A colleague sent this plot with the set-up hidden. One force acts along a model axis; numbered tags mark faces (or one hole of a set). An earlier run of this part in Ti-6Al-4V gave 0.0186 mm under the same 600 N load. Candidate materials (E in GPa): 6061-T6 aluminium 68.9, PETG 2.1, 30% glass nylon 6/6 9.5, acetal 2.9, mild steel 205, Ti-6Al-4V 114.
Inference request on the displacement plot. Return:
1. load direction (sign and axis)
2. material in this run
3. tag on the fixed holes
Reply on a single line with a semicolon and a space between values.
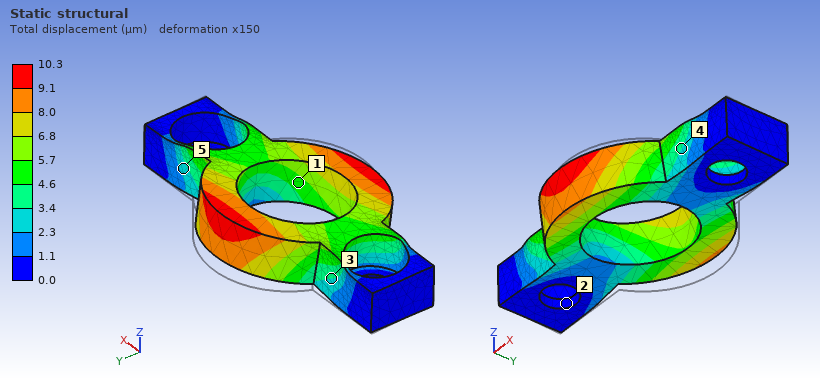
-Y; mild steel; 2
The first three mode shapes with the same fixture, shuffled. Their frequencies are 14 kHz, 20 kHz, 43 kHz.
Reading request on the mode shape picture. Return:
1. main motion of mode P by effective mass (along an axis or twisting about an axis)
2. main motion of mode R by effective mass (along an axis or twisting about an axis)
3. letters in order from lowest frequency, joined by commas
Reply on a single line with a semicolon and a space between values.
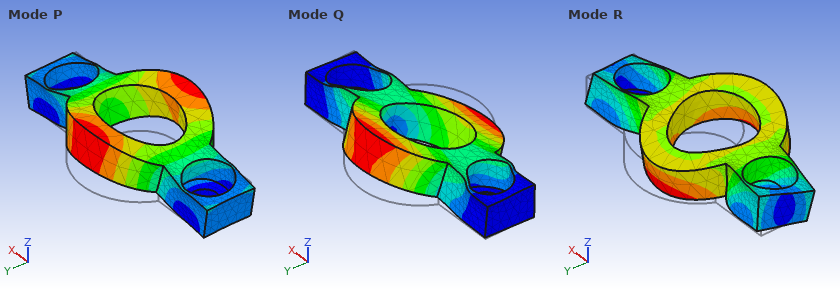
along Z; along Y; Q, P, R
